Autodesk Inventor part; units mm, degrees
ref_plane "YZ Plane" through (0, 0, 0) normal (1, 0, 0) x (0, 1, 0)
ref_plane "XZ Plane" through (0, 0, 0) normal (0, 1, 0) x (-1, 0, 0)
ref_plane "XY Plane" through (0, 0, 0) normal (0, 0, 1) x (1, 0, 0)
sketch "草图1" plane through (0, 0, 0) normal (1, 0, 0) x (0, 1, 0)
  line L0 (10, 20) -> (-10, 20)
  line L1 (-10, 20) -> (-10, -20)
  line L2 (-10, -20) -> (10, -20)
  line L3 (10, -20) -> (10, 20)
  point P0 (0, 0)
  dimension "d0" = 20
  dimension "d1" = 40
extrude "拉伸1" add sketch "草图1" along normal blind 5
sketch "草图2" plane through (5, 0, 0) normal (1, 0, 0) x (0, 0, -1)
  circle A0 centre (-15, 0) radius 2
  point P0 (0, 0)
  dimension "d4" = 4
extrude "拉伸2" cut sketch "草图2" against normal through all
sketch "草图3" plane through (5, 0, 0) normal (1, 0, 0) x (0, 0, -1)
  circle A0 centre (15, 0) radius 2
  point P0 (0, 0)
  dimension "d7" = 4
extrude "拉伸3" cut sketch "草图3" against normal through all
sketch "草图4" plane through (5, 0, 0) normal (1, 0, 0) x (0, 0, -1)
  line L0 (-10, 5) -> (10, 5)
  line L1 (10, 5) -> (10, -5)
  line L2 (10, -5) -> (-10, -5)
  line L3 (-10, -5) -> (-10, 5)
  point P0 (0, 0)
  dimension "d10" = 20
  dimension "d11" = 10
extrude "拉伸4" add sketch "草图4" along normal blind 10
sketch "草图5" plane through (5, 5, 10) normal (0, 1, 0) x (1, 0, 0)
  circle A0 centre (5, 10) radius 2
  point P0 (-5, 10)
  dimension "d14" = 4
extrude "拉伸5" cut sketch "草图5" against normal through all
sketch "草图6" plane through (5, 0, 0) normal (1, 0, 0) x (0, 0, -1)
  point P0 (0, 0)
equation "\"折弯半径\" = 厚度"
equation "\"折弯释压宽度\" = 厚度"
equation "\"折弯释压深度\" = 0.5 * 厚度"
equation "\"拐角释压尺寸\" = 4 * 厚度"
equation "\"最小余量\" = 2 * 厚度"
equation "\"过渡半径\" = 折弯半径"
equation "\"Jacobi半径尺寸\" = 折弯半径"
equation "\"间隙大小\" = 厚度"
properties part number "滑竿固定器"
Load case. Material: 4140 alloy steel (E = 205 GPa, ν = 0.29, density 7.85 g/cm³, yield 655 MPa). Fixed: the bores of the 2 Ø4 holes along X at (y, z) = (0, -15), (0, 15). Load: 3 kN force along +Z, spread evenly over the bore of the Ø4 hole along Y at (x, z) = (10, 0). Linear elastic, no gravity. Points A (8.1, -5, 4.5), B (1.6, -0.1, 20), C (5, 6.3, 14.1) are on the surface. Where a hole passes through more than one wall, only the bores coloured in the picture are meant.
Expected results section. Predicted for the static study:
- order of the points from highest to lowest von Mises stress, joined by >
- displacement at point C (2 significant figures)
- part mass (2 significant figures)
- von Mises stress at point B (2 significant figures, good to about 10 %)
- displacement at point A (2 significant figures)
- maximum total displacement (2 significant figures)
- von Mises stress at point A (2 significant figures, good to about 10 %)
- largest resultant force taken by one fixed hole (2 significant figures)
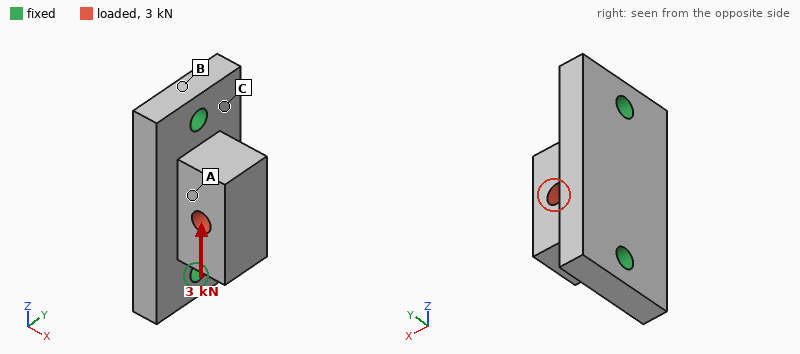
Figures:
A > B > C
0.76 µm
45 g
19 MPa
2.5 µm
4.9 µm
32 MPa
1.7 kN
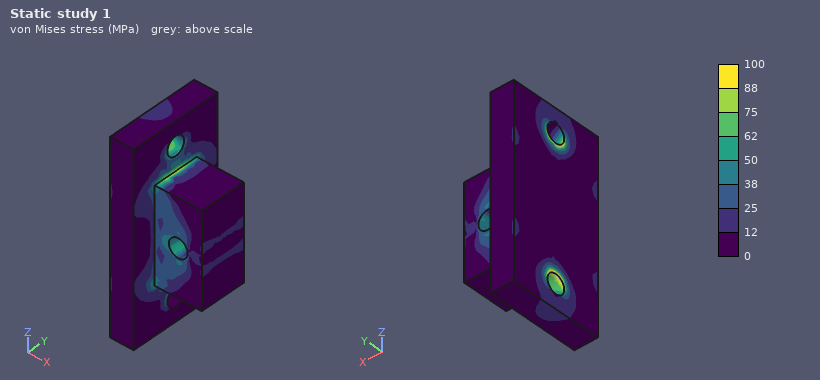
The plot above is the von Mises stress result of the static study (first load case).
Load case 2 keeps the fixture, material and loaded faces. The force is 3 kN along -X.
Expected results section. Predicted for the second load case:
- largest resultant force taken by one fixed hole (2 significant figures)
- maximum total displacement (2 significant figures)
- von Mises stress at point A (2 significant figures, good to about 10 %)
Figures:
1.6 kN
5.7 µm
28 MPa
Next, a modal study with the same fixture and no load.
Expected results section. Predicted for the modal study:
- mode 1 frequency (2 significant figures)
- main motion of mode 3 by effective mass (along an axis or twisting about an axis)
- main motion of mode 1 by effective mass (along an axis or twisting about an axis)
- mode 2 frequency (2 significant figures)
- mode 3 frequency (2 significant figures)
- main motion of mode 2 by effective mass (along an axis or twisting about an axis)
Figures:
15 kHz
along Z
along Y
23 kHz
33 kHz
along X
